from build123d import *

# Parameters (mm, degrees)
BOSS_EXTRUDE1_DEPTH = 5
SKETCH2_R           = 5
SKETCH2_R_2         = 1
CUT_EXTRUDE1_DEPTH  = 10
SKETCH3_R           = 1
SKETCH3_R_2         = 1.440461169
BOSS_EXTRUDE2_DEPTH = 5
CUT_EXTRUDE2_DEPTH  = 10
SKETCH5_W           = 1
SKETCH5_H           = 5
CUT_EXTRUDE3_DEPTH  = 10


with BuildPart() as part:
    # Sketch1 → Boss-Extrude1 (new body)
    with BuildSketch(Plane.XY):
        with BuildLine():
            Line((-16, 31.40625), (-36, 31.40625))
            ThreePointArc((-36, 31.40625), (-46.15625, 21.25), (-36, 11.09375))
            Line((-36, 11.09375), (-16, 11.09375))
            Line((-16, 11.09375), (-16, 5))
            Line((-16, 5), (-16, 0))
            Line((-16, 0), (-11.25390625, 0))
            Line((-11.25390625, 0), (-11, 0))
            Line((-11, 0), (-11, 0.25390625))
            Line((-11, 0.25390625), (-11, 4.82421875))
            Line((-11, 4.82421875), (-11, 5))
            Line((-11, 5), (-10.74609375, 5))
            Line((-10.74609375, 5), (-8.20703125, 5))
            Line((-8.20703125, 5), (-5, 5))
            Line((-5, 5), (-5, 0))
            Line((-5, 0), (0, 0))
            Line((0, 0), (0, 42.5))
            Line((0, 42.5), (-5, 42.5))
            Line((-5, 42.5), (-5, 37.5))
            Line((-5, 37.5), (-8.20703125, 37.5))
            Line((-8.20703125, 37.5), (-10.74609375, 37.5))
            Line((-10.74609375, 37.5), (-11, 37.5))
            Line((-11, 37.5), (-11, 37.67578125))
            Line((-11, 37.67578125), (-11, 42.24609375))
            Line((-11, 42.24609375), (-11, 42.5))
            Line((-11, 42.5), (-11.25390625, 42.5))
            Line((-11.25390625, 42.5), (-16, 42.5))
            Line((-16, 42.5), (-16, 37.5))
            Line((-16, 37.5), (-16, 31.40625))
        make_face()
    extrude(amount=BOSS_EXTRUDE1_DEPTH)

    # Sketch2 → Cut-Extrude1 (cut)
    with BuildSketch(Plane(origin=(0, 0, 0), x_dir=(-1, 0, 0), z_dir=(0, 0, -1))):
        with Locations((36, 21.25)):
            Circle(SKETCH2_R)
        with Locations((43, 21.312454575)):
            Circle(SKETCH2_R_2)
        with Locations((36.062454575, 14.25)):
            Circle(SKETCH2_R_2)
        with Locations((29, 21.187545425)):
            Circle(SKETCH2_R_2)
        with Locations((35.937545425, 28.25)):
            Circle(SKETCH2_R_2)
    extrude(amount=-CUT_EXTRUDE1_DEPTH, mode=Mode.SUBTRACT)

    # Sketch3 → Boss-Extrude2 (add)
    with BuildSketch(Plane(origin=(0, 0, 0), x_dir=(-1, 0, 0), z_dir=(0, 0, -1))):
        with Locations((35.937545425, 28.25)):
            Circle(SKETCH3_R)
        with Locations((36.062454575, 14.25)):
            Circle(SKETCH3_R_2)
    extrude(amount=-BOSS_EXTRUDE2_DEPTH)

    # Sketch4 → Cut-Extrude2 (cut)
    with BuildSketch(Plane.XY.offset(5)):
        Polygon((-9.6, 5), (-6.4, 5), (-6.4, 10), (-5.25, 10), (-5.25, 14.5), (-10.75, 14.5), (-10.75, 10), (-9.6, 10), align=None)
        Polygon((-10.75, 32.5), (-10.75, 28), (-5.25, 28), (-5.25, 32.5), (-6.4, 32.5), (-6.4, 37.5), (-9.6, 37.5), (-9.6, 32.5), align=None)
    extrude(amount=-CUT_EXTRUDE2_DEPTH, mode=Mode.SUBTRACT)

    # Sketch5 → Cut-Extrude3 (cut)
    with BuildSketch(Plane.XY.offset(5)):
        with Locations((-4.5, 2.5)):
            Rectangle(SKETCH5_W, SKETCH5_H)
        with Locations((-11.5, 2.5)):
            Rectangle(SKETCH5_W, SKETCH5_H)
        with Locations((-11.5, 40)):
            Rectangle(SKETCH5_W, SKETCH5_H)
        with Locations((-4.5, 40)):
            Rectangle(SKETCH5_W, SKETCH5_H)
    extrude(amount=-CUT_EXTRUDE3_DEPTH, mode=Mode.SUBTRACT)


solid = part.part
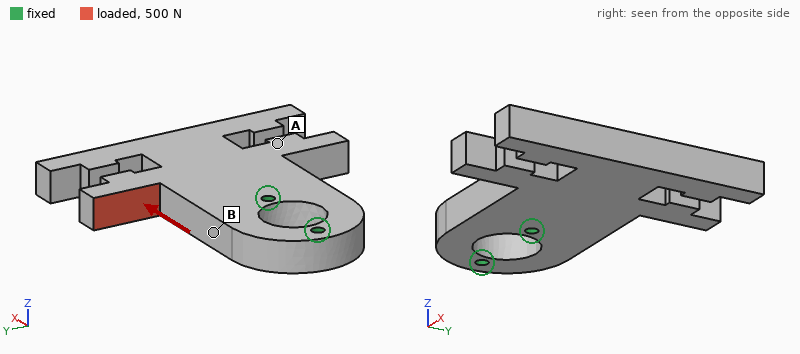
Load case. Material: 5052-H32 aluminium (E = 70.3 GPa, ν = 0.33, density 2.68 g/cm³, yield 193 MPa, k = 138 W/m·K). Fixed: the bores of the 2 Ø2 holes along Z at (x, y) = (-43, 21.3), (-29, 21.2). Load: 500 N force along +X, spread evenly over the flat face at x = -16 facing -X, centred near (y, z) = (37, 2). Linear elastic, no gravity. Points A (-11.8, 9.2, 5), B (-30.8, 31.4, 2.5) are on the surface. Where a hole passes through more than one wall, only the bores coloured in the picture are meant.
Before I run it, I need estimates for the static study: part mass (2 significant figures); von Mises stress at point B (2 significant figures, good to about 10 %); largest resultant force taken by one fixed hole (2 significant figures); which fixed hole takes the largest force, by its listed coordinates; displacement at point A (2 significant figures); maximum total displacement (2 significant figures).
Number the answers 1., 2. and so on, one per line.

1. 13 g
2. 38 MPa
3. 560 N
4. (-29, 21.2)
5. 22 µm
6. 82 µm
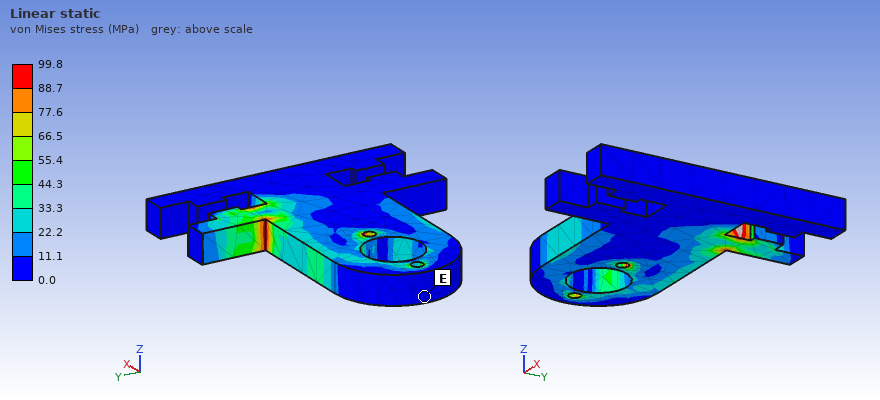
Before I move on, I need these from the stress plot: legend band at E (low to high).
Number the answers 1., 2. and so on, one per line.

1. 0.0 to 11.1 MPa
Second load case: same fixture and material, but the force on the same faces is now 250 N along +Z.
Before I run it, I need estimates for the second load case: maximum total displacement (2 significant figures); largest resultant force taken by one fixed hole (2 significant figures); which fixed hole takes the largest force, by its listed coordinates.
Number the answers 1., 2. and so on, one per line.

1. 0.14 mm
2. 330 N
3. (-29, 21.2)
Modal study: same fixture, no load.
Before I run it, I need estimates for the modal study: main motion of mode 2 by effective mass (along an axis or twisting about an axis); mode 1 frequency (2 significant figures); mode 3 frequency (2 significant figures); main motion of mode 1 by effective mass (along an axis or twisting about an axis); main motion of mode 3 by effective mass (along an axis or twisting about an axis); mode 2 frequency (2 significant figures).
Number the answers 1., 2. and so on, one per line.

1. twisting about X
2. 3300 Hz
3. 6100 Hz
4. along Z
5. along Y
6. 4600 Hz
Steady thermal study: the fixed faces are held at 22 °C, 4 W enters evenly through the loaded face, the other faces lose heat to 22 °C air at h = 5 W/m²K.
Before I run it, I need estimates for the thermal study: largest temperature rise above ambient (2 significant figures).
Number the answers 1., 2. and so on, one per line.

1. 16 K
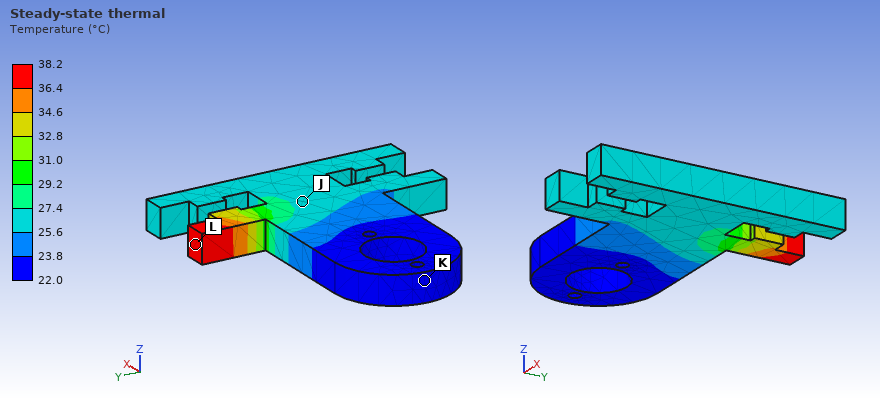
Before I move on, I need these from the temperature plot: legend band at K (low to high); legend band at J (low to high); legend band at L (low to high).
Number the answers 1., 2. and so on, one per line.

1. 22.0 to 23.8 °C
2. 25.6 to 27.4 °C
3. 36.4 to 38.2 °C
